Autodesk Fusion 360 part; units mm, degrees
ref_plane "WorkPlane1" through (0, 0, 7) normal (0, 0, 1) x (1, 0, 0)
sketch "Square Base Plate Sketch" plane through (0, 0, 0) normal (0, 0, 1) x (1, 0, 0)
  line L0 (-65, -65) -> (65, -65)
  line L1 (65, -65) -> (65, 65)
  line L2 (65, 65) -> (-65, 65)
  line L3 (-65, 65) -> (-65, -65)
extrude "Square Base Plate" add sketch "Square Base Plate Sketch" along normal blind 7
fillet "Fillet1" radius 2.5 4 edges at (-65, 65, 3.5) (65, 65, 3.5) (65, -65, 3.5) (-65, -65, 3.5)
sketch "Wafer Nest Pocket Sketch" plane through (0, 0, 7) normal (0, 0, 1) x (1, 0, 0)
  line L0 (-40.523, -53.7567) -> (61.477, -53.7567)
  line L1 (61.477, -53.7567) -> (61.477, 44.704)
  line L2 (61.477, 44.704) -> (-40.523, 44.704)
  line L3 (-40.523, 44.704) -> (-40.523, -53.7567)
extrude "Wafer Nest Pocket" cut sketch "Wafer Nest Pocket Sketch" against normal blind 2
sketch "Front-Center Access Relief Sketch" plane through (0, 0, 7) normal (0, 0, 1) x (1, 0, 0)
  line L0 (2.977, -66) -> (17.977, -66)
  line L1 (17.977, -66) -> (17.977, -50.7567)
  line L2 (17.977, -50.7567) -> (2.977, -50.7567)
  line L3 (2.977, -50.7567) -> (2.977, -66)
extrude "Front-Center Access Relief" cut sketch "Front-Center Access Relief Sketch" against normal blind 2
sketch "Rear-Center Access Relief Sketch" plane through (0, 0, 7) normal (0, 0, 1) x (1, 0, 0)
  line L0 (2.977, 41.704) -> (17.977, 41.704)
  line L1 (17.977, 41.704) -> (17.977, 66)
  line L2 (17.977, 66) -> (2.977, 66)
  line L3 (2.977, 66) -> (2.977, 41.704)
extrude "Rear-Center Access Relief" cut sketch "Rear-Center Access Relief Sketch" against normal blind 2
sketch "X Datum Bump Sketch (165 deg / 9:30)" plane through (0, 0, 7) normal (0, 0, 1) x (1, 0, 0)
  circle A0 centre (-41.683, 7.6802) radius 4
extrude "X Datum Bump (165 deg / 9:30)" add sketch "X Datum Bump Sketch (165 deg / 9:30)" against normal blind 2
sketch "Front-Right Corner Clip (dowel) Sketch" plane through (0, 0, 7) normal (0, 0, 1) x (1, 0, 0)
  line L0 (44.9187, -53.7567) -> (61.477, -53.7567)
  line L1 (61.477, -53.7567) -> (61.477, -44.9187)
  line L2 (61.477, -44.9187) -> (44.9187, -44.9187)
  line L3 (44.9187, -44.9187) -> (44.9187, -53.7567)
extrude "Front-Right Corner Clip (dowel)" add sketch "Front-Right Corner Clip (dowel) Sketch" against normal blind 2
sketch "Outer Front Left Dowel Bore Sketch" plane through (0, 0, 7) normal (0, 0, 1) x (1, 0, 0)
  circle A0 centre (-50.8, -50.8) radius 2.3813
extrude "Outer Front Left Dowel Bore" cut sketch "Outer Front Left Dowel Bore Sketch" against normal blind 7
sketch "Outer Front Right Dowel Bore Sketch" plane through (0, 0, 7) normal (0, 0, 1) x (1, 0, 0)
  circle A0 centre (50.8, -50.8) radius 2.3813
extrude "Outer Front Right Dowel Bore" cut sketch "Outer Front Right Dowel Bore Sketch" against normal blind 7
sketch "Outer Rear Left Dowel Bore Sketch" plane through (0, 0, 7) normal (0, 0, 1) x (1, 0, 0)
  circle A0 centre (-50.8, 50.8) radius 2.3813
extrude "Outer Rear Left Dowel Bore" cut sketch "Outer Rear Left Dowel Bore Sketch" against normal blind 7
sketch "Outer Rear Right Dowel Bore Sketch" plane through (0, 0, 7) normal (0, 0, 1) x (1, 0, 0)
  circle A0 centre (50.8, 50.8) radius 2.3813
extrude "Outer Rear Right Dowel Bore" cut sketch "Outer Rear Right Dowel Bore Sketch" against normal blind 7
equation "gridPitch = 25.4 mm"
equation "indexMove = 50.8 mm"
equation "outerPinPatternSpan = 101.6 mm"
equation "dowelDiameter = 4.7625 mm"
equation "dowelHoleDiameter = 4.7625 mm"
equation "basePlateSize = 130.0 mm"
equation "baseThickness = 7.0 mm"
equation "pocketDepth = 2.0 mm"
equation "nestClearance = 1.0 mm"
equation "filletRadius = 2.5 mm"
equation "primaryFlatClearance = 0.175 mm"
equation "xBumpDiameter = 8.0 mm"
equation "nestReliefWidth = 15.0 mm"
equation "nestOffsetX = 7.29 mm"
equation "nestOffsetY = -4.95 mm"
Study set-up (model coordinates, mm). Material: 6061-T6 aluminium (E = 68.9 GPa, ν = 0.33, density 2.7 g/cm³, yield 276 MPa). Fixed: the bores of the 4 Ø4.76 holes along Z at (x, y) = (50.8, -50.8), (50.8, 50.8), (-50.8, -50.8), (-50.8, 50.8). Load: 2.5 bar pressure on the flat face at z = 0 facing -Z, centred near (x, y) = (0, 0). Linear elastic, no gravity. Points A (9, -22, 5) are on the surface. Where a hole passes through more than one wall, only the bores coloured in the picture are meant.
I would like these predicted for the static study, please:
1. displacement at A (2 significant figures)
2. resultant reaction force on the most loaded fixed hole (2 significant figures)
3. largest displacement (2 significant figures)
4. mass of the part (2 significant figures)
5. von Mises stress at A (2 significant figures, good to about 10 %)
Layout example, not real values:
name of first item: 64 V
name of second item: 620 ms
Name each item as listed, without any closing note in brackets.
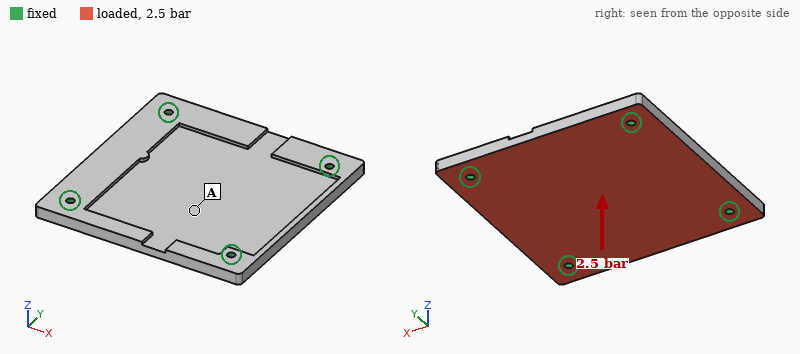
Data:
displacement at A: 0.15 mm
resultant reaction force on the most loaded fixed hole: 1.2 kN
largest displacement: 0.17 mm
mass of the part: 260 g
von Mises stress at A: 23 MPa
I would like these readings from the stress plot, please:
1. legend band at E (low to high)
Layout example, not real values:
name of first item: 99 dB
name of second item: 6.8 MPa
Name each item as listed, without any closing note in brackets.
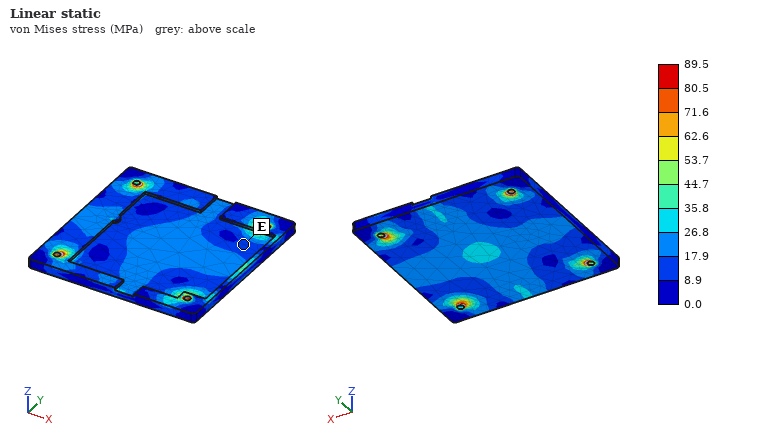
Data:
legend band at E: 8.9 to 17.9 MPa
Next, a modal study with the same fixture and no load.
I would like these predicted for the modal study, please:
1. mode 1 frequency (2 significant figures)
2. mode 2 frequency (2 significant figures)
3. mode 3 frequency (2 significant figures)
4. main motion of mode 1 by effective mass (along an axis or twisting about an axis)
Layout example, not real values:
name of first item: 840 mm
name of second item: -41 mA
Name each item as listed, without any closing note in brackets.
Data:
mode 1 frequency: 2000 Hz
mode 2 frequency: 3100 Hz
mode 3 frequency: 3200 Hz
main motion of mode 1 by effective mass: along Z
